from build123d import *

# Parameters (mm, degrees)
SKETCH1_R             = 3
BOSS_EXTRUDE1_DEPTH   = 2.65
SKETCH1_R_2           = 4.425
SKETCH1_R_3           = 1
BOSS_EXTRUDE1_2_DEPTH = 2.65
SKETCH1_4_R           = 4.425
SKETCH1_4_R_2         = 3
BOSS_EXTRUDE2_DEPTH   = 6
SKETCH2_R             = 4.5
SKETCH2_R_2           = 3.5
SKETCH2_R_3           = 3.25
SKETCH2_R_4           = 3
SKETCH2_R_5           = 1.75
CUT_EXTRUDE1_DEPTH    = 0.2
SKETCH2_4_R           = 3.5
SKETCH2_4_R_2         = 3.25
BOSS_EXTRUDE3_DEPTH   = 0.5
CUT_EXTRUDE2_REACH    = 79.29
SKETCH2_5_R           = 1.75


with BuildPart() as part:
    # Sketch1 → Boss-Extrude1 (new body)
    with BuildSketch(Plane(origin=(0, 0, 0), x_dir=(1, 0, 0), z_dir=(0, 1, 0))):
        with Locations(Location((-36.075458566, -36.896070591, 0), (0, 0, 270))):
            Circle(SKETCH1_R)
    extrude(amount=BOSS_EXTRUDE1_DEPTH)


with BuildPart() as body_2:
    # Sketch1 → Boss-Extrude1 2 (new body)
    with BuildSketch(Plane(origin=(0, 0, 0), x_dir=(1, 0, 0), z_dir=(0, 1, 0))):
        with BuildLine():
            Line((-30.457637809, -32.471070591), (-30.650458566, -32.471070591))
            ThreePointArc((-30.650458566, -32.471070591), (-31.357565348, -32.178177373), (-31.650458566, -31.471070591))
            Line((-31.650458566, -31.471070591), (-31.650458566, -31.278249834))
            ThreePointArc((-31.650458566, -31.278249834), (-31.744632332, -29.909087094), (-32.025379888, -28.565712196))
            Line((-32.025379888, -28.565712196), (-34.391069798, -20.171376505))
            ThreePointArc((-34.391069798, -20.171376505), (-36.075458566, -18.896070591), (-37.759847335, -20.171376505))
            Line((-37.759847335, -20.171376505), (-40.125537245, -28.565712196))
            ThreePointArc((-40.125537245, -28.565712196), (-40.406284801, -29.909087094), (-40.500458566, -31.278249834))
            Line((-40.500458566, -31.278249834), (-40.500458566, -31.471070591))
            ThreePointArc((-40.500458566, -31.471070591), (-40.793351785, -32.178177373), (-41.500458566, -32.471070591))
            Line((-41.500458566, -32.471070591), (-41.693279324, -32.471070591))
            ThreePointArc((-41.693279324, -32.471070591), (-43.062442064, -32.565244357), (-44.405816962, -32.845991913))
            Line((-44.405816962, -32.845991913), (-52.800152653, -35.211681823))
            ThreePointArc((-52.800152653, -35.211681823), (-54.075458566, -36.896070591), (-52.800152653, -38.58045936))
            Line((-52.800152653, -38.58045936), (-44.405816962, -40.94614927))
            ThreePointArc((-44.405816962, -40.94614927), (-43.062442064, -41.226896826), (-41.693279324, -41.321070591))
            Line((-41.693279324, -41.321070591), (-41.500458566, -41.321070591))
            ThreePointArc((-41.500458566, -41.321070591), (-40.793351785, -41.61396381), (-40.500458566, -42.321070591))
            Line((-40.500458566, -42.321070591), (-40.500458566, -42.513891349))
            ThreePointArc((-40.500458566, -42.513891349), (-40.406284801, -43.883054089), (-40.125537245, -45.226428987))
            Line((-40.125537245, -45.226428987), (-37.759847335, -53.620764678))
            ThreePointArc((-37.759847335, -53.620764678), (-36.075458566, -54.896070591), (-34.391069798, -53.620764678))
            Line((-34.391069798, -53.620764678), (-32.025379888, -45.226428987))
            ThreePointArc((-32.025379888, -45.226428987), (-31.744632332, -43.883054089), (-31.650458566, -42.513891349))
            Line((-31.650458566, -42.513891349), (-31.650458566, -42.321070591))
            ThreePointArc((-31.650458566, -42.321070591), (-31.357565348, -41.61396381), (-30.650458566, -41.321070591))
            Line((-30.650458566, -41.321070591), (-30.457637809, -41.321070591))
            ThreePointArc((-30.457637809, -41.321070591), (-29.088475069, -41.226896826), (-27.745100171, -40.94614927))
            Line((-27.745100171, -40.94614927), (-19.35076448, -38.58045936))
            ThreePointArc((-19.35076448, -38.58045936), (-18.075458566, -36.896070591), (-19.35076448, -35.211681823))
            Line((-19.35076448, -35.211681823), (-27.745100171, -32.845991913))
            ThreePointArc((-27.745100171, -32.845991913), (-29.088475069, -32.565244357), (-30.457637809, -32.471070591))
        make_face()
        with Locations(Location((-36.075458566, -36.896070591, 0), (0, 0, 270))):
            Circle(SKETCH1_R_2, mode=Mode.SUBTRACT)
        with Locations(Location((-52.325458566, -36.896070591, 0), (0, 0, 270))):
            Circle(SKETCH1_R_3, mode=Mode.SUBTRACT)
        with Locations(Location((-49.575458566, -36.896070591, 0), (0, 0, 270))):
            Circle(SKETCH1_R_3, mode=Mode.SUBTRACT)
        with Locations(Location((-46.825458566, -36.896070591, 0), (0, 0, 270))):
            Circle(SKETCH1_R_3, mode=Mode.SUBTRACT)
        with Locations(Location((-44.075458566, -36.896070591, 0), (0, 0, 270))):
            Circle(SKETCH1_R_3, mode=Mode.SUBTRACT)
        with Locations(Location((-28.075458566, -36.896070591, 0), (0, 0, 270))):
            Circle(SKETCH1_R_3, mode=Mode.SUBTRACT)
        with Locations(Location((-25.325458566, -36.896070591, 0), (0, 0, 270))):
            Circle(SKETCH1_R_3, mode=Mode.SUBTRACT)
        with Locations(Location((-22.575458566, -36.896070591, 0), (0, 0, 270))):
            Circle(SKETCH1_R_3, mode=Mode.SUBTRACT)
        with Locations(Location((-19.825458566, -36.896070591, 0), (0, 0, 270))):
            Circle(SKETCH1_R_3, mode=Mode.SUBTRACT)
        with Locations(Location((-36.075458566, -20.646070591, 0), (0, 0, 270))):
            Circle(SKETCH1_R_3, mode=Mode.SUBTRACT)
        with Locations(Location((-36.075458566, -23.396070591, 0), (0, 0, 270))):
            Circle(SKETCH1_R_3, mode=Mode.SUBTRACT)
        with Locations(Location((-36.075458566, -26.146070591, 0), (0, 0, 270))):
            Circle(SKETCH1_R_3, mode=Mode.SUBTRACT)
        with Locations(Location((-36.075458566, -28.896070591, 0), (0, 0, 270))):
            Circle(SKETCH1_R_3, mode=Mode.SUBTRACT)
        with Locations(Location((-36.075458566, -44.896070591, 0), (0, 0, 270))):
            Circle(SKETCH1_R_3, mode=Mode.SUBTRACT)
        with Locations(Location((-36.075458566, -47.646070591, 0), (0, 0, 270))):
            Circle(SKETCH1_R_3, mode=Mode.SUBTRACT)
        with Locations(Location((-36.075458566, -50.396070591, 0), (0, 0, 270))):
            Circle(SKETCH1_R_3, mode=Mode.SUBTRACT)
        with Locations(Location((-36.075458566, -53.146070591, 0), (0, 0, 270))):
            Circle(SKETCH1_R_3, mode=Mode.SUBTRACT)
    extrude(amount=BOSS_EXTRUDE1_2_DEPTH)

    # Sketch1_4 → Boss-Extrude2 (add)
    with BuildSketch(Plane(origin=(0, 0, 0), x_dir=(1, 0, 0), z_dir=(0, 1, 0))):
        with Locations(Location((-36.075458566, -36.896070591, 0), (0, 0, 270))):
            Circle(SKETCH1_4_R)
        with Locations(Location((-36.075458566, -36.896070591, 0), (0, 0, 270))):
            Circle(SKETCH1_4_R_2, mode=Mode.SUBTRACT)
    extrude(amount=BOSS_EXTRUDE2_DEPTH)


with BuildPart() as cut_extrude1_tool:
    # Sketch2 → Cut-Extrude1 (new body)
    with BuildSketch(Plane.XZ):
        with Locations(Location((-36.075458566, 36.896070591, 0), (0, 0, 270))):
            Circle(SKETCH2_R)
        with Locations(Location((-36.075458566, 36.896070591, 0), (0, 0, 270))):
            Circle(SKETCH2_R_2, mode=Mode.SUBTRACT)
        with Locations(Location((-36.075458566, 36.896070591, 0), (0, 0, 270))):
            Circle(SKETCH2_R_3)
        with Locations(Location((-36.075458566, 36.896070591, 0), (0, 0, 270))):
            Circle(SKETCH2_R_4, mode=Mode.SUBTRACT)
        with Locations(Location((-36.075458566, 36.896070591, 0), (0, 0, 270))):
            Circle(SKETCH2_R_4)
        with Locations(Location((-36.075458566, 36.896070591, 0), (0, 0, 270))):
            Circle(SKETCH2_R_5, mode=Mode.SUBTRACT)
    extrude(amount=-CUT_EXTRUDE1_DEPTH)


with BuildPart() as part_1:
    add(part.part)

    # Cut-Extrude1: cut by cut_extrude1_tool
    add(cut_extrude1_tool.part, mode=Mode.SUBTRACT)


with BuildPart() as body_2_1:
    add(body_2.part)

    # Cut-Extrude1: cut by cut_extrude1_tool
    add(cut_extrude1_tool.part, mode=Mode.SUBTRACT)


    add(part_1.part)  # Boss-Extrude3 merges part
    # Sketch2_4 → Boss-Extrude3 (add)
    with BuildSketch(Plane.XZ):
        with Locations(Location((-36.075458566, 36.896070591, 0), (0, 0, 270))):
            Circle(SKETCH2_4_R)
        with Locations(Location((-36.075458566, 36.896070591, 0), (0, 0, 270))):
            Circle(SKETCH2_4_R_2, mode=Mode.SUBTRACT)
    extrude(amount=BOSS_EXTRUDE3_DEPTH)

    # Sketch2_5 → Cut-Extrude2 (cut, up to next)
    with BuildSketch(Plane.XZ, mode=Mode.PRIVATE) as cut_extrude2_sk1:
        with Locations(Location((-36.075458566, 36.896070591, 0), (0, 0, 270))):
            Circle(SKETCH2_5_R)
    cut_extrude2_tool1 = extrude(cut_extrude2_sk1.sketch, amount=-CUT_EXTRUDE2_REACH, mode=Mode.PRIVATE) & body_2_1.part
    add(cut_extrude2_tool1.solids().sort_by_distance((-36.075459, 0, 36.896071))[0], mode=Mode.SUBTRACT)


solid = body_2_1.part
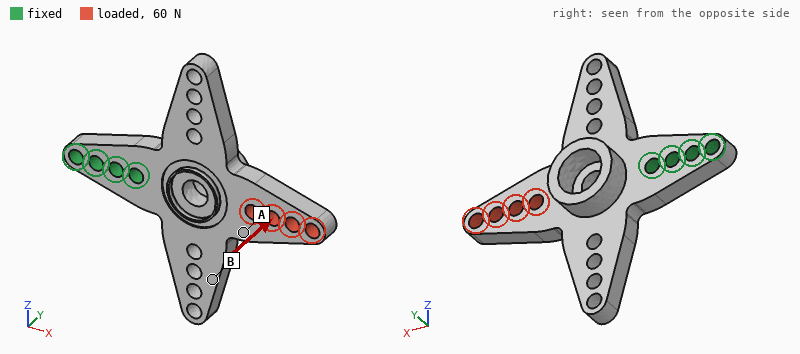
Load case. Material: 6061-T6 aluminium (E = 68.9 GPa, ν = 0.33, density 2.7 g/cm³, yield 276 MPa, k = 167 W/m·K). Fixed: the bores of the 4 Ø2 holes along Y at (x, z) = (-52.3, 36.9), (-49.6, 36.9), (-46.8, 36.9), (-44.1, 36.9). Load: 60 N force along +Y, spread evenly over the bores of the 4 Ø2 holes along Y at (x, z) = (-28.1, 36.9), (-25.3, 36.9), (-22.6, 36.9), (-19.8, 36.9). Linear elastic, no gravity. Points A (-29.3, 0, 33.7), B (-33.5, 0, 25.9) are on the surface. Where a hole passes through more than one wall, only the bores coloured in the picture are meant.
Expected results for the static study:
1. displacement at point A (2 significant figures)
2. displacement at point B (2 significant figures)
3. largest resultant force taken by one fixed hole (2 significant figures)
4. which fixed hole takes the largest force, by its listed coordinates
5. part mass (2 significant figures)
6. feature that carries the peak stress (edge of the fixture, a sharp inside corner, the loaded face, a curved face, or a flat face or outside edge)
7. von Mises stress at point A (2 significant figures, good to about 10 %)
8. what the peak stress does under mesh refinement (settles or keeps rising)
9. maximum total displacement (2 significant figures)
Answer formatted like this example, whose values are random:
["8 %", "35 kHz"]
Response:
["0.089 mm", "0.048 mm", "160 N", "(-44.1, 36.9)", "2.9 g", "edge of the fixture", "38 MPa", "keeps rising", "0.21 mm"]
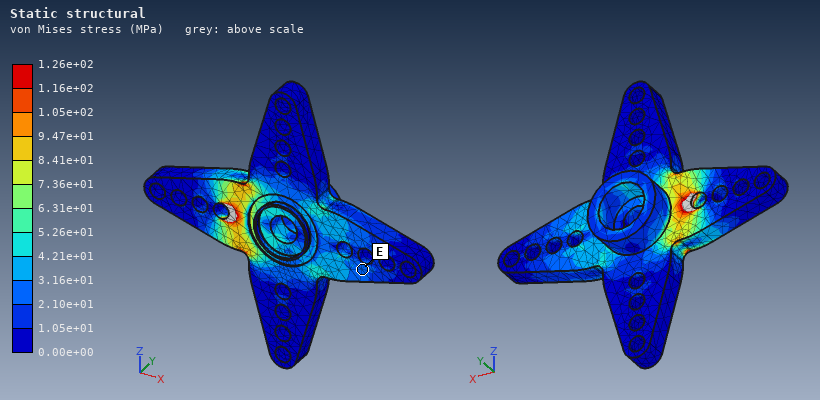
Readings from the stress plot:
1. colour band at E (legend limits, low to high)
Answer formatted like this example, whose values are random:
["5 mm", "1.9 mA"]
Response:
["2.10e+01 to 3.16e+01 MPa"]
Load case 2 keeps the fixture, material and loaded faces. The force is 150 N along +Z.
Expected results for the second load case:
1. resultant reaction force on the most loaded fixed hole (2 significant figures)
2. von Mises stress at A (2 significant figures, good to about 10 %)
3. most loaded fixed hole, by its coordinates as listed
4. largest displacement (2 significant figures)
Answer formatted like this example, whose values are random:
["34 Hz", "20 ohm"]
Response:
["560 N", "23 MPa", "(-44.1, 36.9)", "87 µm"]
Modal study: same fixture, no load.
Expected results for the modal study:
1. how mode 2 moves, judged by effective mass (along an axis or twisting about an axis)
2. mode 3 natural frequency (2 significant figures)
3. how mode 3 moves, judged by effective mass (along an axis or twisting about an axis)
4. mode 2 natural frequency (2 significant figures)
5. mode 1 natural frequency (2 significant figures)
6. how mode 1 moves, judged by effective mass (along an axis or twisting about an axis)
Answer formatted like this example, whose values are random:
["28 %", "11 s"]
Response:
["twisting about X", "8100 Hz", "along Z", "6600 Hz", "4500 Hz", "along Y"]
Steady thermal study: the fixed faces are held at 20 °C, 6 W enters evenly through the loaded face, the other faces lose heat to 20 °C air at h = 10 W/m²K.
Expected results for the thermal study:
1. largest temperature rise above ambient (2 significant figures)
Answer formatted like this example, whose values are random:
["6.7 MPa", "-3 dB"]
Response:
["35 K"]
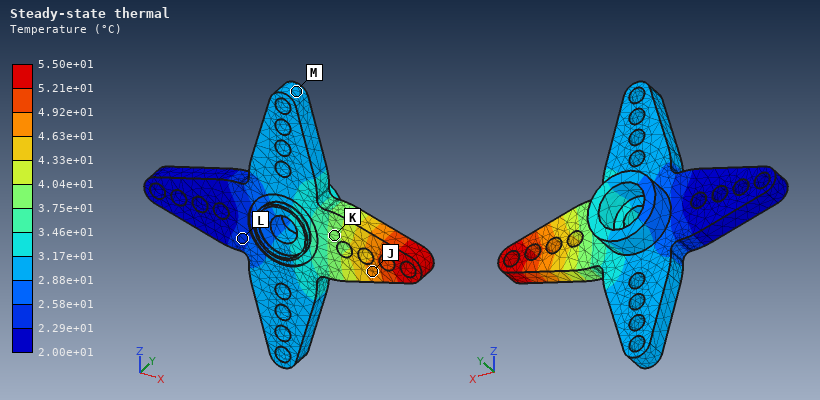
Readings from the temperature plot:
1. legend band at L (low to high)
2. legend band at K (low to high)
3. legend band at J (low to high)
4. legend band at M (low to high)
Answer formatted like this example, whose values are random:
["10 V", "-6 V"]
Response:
["2.29e+01 to 2.58e+01 °C", "3.75e+01 to 4.04e+01 °C", "4.63e+01 to 4.92e+01 °C", "2.88e+01 to 3.17e+01 °C"]
